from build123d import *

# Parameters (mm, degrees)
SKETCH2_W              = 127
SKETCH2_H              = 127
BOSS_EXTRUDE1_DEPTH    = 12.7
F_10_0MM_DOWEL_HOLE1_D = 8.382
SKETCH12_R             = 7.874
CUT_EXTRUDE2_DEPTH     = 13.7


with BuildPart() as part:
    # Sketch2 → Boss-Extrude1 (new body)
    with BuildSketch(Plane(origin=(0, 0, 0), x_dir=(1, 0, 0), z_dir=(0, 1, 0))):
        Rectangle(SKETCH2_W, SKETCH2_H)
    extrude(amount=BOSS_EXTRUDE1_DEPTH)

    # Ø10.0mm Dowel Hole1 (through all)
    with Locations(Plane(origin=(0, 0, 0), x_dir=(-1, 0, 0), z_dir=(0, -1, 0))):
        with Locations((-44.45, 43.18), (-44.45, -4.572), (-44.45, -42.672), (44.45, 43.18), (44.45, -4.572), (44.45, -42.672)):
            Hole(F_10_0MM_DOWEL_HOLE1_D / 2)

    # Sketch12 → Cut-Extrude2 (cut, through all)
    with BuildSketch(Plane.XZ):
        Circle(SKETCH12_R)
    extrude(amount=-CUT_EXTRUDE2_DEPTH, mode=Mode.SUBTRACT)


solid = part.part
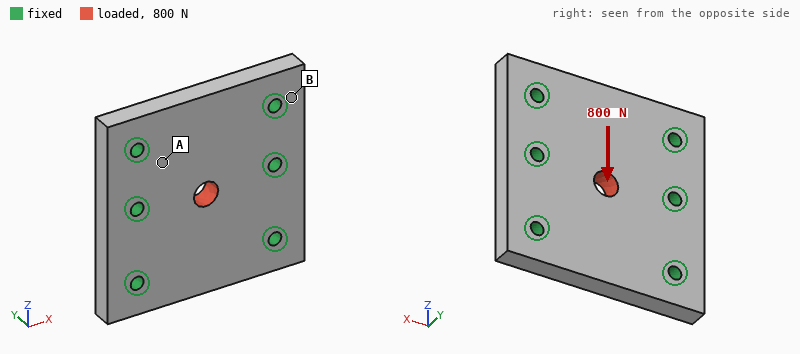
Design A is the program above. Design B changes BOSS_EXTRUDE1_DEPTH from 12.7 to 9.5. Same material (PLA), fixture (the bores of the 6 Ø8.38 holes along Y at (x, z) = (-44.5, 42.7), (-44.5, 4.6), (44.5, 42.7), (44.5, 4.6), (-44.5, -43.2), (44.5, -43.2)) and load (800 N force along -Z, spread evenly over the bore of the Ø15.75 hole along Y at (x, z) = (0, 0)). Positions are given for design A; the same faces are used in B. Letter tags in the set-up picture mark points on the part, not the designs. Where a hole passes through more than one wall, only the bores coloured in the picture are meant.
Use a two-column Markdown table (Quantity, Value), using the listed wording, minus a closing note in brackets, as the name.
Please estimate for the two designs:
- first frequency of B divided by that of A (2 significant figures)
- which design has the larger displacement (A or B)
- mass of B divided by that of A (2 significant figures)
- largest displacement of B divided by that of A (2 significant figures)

| Quantity | Value |
|---|---|
| first frequency of B divided by that of A | 0.81 |
| which design has the larger displacement | B |
| mass of B divided by that of A | 0.75 |
| largest displacement of B divided by that of A | 1.3 |
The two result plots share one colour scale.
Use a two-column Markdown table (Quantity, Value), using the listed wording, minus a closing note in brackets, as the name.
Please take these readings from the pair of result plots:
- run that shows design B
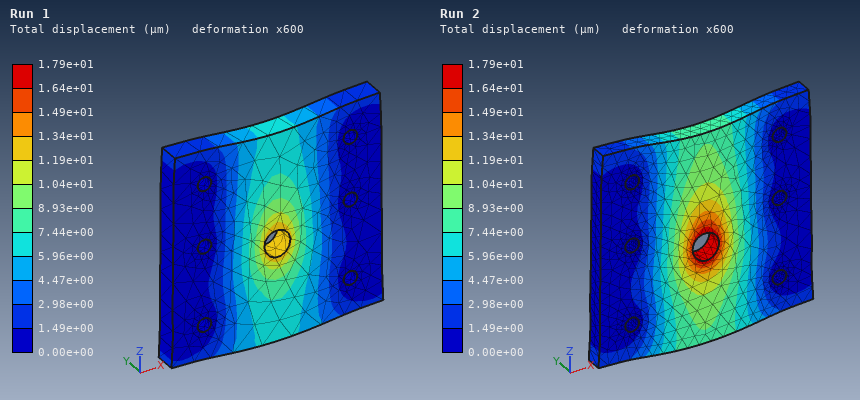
| Quantity | Value |
|---|---|
| run that shows design B | Run 2 |
